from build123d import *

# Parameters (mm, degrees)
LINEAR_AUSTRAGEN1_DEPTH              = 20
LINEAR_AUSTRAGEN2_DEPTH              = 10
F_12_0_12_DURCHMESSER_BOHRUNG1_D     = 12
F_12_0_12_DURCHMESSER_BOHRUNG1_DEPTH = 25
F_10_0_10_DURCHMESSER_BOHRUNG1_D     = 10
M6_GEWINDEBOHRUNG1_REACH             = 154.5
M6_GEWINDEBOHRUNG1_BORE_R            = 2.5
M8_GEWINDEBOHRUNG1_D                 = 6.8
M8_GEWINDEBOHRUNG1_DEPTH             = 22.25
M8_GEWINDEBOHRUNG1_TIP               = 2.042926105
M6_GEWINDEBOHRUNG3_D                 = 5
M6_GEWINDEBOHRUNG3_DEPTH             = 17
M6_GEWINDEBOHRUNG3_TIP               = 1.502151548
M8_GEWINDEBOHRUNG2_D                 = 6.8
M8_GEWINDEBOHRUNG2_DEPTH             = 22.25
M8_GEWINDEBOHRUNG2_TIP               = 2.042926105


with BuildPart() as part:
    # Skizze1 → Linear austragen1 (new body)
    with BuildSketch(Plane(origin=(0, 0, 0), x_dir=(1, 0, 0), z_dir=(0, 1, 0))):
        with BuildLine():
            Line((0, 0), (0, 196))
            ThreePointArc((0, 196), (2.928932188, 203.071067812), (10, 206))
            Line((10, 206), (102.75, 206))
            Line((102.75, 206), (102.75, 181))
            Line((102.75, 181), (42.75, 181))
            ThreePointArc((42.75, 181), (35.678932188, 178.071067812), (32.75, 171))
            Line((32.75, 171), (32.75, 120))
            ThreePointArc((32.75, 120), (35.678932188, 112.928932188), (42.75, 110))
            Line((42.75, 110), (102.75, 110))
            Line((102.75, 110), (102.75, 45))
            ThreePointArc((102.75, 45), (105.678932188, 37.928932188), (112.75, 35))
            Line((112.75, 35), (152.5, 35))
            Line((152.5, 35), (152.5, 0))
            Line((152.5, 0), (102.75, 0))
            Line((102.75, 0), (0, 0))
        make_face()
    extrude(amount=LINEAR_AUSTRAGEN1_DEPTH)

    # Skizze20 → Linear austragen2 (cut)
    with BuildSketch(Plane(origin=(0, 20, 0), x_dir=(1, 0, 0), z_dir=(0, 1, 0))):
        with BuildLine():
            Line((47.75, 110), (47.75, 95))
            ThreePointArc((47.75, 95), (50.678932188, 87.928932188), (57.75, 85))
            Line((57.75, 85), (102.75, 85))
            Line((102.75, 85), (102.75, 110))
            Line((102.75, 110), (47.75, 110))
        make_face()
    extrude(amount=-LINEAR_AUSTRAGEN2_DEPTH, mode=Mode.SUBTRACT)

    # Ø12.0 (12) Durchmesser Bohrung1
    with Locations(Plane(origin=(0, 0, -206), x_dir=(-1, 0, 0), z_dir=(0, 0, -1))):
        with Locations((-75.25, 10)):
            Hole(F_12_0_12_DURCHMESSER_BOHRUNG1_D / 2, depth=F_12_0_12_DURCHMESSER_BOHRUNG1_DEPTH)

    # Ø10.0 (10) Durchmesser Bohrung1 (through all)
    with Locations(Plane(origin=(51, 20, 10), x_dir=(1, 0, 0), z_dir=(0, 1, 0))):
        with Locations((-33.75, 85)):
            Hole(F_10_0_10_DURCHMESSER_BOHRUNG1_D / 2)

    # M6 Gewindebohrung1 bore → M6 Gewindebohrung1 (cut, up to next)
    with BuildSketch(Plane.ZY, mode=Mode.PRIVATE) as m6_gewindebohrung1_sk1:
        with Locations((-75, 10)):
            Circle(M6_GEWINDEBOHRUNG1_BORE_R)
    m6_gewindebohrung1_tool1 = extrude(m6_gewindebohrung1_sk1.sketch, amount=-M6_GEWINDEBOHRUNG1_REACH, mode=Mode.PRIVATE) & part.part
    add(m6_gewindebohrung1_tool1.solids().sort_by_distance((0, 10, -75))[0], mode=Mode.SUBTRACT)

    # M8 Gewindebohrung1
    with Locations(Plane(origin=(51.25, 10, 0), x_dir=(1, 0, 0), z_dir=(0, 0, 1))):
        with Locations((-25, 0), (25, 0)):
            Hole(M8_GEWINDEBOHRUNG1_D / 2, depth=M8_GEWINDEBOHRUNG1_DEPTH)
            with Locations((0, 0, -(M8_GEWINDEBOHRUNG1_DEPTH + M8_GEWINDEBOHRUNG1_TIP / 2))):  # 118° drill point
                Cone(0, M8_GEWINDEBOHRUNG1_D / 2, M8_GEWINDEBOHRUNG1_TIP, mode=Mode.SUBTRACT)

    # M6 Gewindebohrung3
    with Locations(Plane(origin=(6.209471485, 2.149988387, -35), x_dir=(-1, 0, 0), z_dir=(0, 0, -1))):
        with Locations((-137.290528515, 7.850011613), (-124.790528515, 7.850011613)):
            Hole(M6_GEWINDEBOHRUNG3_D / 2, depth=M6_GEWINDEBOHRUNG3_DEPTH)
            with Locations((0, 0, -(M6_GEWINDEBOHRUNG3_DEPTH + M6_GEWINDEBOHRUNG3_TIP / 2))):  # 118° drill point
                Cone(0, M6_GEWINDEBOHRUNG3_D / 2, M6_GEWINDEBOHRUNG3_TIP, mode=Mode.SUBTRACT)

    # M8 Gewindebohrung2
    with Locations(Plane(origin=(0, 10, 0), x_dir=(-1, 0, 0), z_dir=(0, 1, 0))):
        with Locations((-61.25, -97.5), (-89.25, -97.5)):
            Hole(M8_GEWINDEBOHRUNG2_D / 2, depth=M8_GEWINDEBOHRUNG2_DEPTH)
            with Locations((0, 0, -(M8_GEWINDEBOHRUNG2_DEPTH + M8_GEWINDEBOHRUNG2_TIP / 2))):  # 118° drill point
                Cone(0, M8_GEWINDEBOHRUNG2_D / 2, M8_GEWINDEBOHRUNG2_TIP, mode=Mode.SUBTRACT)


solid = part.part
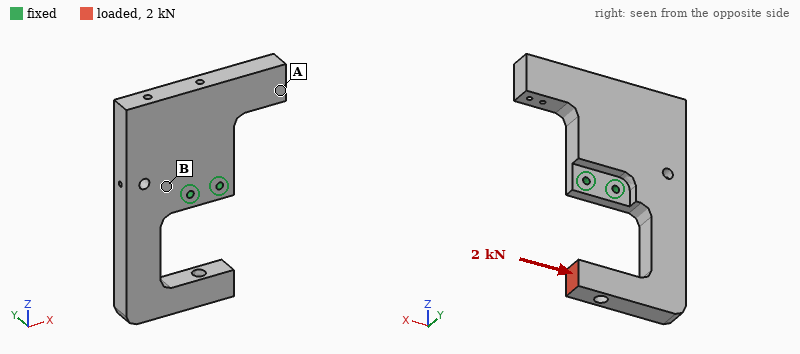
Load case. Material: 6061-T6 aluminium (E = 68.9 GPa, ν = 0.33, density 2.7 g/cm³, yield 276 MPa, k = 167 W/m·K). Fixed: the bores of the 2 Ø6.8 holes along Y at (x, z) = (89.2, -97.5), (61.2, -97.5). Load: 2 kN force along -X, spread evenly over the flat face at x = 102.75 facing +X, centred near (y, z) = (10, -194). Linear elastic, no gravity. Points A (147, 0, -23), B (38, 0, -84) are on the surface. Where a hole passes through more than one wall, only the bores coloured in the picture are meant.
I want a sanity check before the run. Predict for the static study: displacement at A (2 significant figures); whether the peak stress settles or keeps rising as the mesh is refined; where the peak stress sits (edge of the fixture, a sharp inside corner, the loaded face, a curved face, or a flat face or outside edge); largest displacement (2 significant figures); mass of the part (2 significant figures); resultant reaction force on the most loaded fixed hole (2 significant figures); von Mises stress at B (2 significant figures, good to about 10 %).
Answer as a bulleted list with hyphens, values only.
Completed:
- 0.081 mm
- keeps rising
- edge of the fixture
- 0.39 mm
- 910 g
- 6.3 kN
- 15 MPa
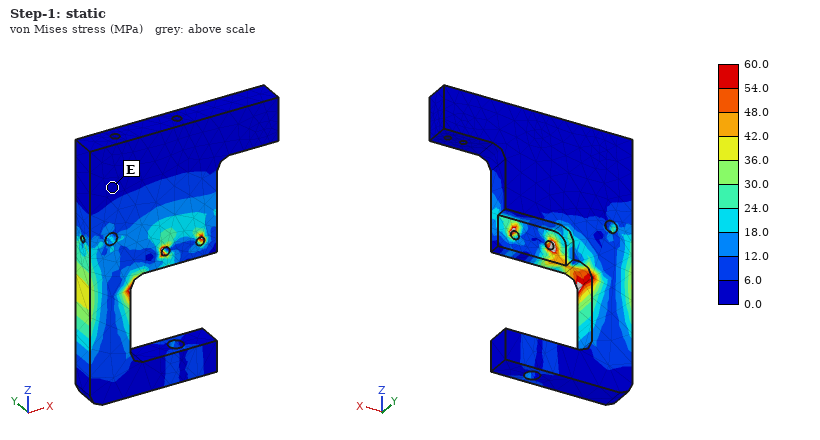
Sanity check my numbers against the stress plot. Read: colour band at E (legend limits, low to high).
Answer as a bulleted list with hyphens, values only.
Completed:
- 0.0 to 6.0 MPa
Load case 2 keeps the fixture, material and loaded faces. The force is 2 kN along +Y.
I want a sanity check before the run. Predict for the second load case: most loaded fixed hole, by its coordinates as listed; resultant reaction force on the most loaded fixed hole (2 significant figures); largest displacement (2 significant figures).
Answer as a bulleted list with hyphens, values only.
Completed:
- (89.2, -97.5)
- 2.4 kN
- 2.8 mm
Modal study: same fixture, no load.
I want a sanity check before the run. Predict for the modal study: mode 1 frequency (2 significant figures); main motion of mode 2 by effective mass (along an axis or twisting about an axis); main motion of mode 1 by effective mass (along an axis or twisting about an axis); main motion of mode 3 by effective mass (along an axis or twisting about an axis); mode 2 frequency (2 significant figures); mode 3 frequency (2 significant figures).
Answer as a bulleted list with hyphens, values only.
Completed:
- 410 Hz
- along Y
- twisting about X
- along Y
- 830 Hz
- 900 Hz
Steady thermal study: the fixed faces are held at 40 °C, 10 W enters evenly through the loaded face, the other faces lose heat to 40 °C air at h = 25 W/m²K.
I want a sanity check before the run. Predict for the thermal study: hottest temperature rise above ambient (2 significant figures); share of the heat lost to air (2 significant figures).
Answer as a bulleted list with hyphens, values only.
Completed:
- 17 K
- 44 %
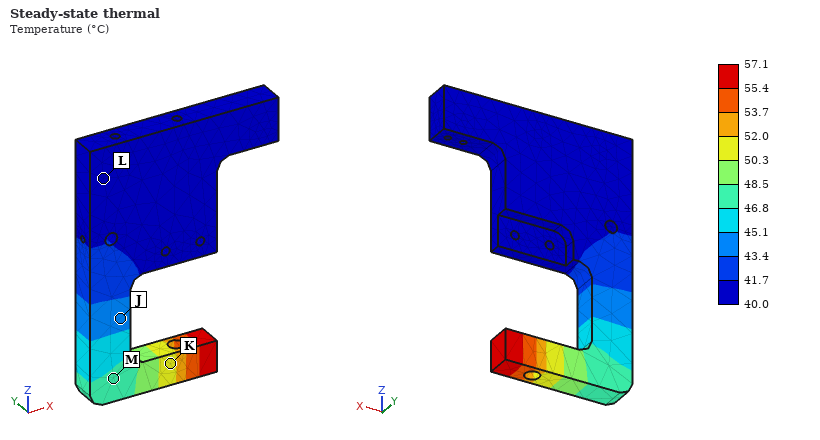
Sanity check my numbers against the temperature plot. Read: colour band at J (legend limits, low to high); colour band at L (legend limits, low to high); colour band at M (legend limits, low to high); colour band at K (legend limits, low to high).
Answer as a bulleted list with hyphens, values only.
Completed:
- 43.4 to 45.1 °C
- 40.0 to 41.7 °C
- 46.8 to 48.5 °C
- 50.3 to 52.0 °C
